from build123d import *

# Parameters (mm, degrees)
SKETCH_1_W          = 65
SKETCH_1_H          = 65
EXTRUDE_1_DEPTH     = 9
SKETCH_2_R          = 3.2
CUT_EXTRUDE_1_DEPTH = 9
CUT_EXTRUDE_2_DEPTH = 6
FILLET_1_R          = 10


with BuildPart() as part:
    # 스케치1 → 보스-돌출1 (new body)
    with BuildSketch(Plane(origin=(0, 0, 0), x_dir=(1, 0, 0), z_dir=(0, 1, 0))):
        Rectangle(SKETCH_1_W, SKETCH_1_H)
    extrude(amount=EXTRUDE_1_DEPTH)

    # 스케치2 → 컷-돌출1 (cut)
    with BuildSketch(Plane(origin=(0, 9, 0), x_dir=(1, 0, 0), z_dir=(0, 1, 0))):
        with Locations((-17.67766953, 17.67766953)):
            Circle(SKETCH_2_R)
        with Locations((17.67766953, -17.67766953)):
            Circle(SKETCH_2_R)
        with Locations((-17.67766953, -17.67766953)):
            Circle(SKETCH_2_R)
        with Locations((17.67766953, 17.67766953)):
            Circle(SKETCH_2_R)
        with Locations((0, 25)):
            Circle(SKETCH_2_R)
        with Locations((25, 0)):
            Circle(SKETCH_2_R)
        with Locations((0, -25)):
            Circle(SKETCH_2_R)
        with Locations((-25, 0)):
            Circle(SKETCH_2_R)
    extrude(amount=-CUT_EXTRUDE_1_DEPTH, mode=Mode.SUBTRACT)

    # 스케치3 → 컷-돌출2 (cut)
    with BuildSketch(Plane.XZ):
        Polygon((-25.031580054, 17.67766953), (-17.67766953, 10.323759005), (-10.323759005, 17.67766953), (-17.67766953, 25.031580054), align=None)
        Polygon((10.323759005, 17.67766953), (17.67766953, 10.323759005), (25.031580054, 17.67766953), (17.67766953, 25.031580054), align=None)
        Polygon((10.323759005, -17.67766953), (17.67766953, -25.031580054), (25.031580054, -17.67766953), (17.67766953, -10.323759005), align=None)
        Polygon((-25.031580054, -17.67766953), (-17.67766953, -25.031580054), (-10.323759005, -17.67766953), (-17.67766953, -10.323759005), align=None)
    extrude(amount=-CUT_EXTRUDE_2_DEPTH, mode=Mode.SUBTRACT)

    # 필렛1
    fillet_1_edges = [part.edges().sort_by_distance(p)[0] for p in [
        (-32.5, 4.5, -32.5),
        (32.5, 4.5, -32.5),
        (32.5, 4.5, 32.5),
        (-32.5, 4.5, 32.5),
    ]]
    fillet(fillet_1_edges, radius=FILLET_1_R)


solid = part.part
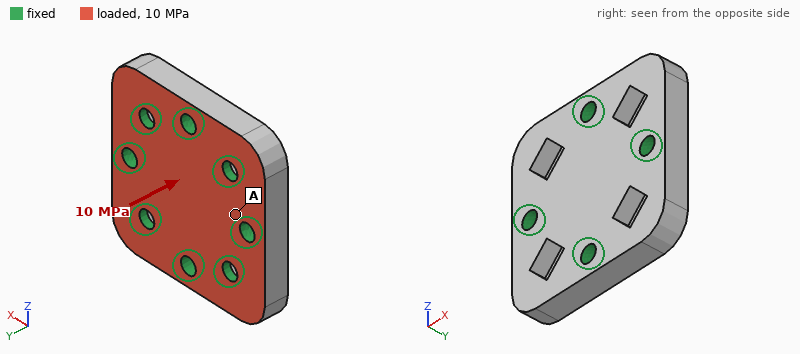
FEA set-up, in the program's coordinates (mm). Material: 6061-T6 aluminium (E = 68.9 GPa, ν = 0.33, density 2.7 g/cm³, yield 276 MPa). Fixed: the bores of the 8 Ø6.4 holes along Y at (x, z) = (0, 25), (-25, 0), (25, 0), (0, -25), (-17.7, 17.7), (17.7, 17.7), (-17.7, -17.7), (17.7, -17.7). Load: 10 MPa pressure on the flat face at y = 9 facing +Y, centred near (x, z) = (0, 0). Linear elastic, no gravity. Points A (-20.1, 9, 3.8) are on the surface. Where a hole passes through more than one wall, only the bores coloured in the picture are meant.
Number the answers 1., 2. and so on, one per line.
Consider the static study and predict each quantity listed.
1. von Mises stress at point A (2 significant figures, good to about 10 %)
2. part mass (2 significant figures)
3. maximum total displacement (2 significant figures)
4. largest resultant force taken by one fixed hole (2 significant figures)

1. 36 MPa
2. 89 g
3. 39 µm
4. 5.5 kN
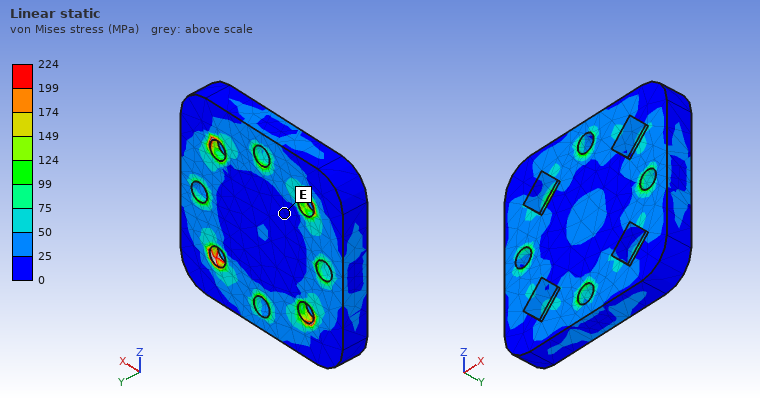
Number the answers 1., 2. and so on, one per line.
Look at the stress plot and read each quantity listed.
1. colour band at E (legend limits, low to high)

1. 0 to 25 MPa
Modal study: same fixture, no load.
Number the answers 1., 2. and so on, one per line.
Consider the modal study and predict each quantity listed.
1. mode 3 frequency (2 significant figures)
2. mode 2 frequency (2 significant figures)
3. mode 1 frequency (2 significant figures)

1. 20 kHz
2. 20 kHz
3. 20 kHz
